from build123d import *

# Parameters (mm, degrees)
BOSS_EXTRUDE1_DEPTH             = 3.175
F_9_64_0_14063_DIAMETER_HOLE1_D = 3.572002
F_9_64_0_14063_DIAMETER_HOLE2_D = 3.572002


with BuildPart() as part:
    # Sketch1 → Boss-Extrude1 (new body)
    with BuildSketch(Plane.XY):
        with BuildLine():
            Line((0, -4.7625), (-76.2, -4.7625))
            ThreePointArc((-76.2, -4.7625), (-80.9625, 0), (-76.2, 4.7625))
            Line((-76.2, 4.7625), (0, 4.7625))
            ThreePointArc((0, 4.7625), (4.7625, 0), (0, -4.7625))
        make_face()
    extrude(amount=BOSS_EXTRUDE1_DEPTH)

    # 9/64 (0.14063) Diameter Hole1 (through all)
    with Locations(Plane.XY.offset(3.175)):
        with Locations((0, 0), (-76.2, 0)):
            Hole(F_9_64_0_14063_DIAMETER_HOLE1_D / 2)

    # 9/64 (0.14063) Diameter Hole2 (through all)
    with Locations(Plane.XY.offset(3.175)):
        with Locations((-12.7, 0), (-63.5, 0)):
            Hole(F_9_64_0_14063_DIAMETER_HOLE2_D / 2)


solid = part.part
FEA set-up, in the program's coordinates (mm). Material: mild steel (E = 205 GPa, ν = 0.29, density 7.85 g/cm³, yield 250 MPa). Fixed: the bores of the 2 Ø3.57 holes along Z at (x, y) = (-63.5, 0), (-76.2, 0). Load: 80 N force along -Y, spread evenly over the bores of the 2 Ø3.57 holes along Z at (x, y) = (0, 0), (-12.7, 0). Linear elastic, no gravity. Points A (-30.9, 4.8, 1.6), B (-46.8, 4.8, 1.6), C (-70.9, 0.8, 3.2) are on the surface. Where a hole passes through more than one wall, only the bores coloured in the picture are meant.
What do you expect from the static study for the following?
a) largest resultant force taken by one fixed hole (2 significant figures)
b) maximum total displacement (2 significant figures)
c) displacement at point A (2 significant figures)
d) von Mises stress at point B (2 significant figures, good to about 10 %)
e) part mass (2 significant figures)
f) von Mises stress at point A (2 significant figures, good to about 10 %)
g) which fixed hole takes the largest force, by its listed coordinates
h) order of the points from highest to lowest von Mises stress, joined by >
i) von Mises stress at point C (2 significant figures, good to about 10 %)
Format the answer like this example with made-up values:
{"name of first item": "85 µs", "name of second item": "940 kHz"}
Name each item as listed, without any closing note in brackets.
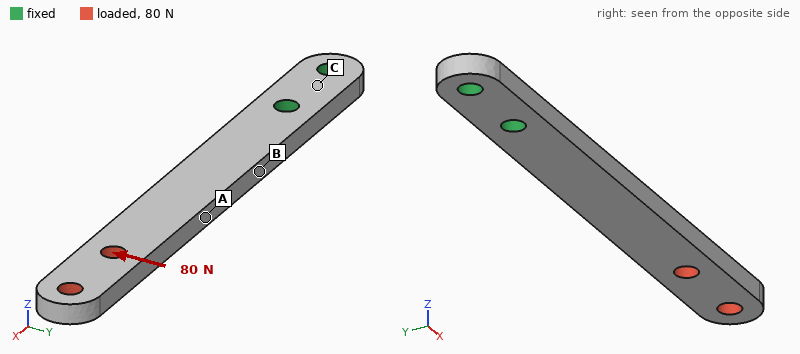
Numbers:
{"largest resultant force taken by one fixed hole": "220 N", "maximum total displacement": "0.15 mm", "displacement at point A": "0.051 mm", "von Mises stress at point B": "67 MPa", "part mass": "19 g", "von Mises stress at point A": "41 MPa", "which fixed hole takes the largest force, by its listed coordinates": "(-63.5, 0)", "order of the points from highest to lowest von Mises stress, joined by >": "B > A > C", "von Mises stress at point C": "11 MPa"}
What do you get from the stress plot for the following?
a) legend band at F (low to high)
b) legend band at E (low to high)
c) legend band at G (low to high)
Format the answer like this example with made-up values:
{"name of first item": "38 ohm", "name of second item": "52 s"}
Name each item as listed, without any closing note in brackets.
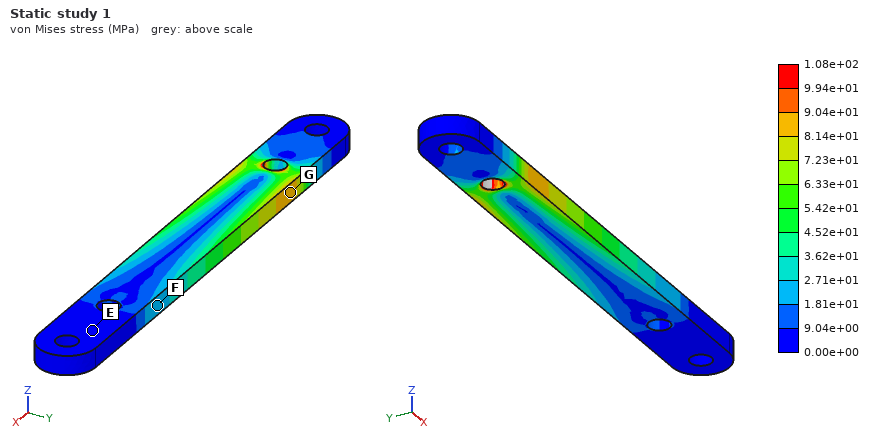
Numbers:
{"legend band at F": "1.81e+01 to 2.71e+01 MPa", "legend band at E": "0.00e+00 to 9.04e+00 MPa", "legend band at G": "8.14e+01 to 9.04e+01 MPa"}
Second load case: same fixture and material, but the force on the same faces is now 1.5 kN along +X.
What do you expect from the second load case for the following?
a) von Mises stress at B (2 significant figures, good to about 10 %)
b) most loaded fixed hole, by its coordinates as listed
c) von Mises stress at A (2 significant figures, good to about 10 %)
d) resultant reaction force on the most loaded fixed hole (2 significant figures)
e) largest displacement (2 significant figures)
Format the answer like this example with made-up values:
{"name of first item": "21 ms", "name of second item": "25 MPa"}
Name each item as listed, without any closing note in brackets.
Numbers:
{"von Mises stress at B": "50 MPa", "most loaded fixed hole, by its coordinates as listed": "(-63.5, 0)", "von Mises stress at A": "50 MPa", "resultant reaction force on the most loaded fixed hole": "1.4 kN", "largest displacement": "15 µm"}
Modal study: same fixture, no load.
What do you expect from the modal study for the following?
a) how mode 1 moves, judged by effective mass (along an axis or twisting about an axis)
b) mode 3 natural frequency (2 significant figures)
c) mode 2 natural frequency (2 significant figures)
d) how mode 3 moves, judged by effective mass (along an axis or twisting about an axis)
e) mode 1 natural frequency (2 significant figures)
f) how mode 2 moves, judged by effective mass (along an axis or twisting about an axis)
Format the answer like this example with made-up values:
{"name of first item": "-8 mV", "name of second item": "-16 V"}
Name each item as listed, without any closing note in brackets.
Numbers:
{"how mode 1 moves, judged by effective mass": "along Z", "mode 3 natural frequency": "3700 Hz", "mode 2 natural frequency": "1700 Hz", "how mode 3 moves, judged by effective mass": "along Z", "mode 1 natural frequency": "620 Hz", "how mode 2 moves, judged by effective mass": "along Y"}
